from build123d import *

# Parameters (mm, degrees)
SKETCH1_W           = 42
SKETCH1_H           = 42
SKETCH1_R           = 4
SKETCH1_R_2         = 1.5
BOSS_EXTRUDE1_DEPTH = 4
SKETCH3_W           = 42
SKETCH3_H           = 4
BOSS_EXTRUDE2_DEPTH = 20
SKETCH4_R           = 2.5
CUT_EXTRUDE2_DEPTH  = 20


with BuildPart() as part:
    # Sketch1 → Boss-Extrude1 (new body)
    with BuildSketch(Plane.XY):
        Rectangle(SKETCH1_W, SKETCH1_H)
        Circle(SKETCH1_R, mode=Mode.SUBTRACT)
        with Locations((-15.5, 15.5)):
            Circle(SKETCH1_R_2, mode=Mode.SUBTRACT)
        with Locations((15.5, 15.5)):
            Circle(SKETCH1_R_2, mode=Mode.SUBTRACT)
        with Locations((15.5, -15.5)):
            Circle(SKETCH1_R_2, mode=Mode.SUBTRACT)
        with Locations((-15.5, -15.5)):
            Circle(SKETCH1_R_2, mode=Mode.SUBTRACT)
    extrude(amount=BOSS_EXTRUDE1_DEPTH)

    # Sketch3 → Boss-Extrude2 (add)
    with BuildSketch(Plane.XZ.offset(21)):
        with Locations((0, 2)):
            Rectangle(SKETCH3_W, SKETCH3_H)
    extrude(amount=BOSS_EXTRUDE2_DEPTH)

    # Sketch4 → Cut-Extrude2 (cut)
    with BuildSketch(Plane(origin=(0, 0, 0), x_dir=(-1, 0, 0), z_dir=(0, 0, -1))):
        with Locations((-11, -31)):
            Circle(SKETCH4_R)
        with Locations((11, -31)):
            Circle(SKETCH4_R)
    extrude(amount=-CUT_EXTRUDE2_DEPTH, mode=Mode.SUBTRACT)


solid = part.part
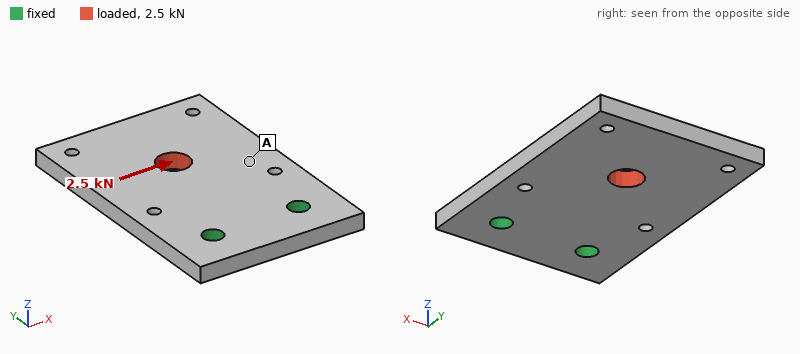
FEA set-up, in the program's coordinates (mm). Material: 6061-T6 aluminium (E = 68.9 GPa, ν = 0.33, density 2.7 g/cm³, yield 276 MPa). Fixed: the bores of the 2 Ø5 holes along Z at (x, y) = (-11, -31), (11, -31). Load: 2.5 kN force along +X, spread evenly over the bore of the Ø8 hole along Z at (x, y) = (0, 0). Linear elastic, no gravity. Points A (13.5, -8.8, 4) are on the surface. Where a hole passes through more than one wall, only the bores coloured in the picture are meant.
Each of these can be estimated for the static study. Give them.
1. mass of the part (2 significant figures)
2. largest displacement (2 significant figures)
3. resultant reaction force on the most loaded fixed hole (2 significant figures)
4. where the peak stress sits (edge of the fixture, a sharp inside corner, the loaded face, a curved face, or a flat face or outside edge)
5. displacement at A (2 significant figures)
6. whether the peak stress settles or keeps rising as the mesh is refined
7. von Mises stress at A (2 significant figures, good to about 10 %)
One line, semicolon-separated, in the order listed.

27 g; 72 µm; 3.3 kN; edge of the fixture; 33 µm; keeps rising; 22 MPa
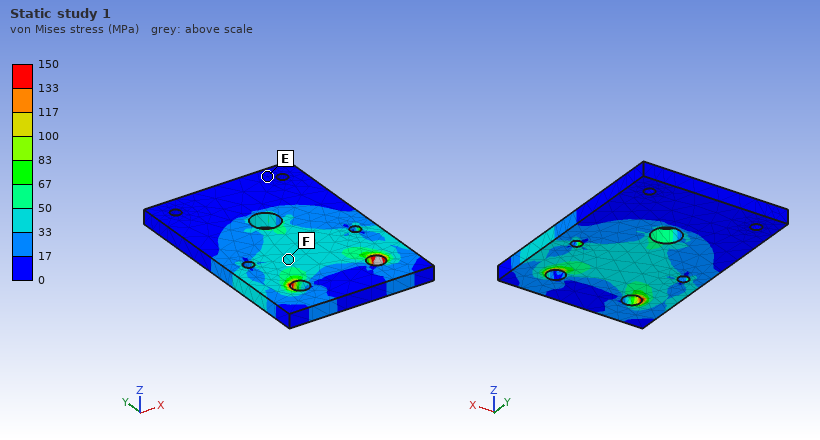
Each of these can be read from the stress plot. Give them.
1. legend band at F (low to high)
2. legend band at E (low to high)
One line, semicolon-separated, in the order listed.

33 to 50 MPa; 0 to 17 MPa
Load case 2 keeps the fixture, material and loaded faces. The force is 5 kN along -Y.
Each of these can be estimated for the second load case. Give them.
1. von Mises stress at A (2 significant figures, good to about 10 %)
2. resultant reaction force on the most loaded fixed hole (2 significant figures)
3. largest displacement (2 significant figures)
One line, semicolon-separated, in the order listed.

23 MPa; 2.5 kN; 24 µm
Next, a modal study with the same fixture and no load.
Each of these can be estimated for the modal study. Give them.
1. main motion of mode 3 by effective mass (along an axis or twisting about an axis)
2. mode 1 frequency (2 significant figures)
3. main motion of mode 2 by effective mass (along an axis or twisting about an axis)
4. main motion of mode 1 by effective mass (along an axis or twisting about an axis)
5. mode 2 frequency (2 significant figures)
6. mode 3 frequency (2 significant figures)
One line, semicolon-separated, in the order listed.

along Z; 1300 Hz; twisting about Y; along Z; 3400 Hz; 7400 Hz
